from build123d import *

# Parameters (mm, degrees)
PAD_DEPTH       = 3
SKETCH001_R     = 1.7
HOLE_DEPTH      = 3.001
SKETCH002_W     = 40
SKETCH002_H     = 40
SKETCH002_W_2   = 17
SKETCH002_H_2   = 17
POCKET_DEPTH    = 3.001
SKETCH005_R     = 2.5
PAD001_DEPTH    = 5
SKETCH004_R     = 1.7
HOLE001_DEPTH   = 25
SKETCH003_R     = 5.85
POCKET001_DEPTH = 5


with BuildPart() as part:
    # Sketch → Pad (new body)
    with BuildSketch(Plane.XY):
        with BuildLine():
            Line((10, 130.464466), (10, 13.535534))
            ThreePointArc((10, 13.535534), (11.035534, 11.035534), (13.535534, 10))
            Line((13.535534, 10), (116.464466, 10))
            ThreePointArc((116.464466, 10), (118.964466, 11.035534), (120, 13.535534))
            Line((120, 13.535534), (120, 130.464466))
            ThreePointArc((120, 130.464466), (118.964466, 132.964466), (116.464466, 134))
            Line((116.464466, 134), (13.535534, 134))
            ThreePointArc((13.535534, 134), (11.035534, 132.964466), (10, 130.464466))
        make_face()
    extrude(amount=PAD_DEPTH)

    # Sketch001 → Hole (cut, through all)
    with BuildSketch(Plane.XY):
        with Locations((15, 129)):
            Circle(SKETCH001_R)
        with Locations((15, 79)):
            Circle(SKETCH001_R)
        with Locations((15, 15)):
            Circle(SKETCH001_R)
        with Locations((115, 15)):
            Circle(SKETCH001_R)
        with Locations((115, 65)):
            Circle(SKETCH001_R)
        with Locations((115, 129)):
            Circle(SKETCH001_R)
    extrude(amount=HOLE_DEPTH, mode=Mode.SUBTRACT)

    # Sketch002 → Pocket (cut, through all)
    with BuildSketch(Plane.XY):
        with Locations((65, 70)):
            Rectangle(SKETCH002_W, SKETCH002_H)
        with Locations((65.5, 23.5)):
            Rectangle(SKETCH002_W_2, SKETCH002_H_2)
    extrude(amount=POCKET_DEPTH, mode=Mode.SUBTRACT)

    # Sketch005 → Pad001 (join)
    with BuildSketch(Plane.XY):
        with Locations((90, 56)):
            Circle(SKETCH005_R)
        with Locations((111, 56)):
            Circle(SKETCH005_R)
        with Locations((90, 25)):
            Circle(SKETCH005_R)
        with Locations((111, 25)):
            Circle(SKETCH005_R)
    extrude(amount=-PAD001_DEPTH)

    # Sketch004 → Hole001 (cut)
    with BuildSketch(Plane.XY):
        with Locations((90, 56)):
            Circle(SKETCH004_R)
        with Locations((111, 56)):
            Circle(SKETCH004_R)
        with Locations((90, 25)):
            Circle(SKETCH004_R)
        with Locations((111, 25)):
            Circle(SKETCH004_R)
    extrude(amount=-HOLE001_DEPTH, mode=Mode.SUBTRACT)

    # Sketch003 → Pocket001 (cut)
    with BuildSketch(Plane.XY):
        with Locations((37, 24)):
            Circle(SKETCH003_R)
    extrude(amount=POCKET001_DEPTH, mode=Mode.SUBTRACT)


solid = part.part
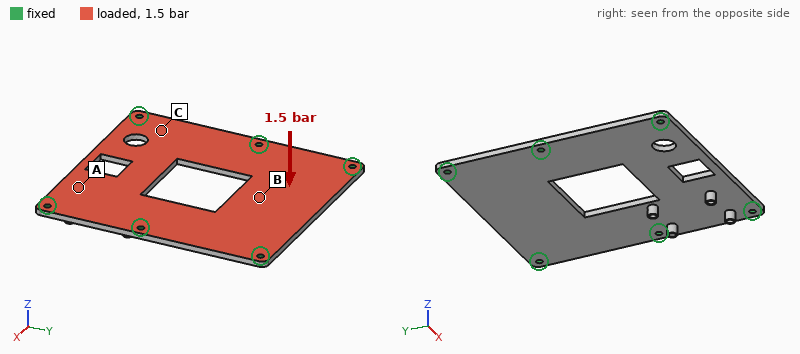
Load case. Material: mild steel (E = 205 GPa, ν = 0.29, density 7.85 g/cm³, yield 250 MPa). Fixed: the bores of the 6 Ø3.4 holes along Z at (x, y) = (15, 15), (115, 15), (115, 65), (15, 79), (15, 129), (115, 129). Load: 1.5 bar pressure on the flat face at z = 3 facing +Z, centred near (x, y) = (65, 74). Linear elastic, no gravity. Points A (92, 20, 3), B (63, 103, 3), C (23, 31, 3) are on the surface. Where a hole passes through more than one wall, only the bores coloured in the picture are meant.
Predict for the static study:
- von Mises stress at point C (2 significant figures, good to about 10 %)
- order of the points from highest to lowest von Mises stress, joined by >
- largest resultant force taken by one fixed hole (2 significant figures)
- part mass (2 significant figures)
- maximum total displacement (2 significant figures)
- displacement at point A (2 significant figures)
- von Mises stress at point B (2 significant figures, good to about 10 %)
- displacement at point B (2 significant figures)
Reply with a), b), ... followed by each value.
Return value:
a) 25 MPa
b) B > C > A
c) 410 N
d) 270 g
e) 0.13 mm
f) 0.060 mm
g) 44 MPa
h) 0.12 mm
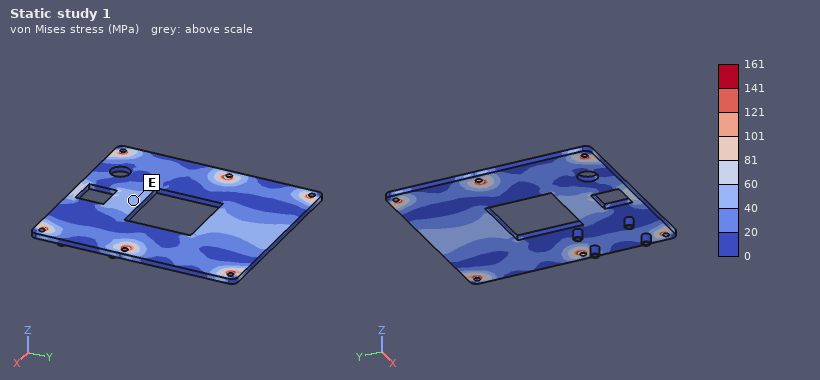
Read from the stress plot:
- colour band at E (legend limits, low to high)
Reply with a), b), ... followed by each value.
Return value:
a) 40 to 60 MPa
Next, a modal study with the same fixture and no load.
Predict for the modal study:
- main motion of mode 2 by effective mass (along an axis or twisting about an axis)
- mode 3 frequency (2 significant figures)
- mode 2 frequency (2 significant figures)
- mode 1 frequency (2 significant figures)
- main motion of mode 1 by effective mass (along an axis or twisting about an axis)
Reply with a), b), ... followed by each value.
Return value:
a) twisting about X
b) 2700 Hz
c) 1500 Hz
d) 1300 Hz
e) along Z
